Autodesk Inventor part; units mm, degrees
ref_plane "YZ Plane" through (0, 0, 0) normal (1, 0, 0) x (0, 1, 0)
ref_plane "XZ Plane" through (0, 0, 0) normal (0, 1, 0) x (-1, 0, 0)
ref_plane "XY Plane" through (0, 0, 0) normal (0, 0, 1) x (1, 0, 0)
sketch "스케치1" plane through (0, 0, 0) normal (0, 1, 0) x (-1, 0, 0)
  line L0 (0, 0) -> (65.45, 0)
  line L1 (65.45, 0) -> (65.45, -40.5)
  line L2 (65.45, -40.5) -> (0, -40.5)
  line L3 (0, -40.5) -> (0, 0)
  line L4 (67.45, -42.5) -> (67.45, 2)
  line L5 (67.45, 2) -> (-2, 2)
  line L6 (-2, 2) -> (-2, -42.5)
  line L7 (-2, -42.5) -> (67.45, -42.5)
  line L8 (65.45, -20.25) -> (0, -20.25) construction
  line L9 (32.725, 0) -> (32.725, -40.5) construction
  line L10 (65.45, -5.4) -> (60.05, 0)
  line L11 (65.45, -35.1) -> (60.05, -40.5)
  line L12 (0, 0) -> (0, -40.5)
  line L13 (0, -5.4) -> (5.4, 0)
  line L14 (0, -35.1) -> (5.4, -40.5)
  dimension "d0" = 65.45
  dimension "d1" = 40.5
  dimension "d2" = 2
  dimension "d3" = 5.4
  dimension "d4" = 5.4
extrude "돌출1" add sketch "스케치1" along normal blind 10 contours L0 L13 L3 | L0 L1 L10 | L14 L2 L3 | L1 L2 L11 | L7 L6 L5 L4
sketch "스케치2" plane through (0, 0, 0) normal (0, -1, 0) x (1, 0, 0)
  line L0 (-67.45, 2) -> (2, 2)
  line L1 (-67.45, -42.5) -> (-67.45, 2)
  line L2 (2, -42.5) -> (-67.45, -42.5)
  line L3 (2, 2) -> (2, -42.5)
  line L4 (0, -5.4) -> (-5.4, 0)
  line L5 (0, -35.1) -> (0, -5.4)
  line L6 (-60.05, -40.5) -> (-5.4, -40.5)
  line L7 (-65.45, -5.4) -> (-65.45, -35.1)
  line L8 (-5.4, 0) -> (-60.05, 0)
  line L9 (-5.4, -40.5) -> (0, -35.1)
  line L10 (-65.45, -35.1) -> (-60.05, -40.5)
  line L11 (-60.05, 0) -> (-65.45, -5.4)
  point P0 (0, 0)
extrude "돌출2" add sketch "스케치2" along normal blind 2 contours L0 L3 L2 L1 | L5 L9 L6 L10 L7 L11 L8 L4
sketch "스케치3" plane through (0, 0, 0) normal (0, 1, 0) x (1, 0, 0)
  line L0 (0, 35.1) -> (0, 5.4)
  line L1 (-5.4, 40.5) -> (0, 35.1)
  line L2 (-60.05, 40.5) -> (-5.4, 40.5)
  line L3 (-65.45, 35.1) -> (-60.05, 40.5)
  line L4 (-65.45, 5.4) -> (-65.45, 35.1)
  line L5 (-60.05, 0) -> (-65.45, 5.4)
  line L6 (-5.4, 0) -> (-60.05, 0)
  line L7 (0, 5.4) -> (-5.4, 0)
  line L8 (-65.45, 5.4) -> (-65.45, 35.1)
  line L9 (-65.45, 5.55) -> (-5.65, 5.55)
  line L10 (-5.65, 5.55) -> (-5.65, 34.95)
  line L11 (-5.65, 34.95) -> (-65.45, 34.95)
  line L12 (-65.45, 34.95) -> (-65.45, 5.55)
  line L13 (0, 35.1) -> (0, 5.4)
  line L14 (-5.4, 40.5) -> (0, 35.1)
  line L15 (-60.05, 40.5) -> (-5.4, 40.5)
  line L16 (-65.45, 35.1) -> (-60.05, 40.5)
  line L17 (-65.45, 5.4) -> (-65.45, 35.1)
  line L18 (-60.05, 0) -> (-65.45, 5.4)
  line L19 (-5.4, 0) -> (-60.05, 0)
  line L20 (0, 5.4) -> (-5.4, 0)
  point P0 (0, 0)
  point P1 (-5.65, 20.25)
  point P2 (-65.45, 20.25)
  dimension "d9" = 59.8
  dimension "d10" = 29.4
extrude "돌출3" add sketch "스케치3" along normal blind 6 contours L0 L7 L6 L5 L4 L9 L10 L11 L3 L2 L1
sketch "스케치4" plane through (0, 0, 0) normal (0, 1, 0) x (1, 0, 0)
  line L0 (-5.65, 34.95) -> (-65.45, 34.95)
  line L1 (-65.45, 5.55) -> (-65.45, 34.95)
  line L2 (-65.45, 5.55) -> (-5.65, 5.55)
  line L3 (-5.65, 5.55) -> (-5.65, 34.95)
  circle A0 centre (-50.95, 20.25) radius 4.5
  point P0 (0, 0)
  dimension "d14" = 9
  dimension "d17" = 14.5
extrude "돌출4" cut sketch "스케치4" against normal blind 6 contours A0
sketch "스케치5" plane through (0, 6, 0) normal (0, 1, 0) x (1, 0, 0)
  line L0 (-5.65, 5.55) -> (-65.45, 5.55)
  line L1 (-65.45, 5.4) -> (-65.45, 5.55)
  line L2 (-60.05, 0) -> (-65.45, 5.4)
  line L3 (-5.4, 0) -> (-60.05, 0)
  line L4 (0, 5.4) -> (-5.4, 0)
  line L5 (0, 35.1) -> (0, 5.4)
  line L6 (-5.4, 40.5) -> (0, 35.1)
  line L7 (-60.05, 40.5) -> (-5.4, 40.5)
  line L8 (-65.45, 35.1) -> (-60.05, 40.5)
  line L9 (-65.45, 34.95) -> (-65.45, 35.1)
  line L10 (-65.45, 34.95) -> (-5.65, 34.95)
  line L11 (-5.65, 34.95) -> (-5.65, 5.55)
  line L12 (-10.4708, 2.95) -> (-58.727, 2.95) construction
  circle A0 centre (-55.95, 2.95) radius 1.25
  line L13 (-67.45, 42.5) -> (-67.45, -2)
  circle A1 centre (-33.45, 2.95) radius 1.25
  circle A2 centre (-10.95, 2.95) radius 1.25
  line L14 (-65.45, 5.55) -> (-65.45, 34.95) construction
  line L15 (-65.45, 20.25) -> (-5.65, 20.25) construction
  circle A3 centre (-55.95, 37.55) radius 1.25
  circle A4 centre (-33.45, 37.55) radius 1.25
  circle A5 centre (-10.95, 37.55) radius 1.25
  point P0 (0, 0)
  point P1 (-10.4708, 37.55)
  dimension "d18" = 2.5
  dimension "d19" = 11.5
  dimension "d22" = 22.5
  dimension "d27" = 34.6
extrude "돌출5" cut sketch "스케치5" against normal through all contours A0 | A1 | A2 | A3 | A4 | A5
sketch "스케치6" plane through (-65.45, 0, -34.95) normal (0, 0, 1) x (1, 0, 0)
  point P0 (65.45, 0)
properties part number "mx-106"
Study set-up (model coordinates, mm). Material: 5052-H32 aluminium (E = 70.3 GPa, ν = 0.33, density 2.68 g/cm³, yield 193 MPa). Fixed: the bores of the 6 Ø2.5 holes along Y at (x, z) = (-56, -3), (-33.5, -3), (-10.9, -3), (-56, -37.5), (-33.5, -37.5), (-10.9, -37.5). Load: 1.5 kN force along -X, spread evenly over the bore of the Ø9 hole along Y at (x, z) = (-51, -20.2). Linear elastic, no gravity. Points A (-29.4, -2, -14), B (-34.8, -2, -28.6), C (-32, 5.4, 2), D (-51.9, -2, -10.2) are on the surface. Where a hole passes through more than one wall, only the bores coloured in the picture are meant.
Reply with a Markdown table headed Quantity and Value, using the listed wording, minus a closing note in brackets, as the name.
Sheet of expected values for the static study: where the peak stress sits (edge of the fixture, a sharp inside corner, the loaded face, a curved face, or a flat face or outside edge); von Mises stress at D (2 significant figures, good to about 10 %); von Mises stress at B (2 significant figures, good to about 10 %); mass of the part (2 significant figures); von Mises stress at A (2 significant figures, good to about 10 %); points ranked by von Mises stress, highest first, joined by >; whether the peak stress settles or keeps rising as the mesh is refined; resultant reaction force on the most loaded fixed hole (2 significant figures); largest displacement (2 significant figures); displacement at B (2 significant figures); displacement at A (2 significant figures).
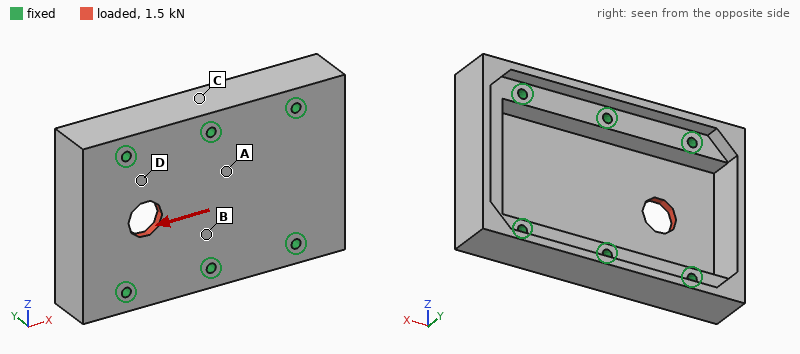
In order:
| Quantity | Value |
|---|---|
| where the peak stress sits | a sharp inside corner |
| von Mises stress at D | 16 MPa |
| von Mises stress at B | 11 MPa |
| mass of the part | 42 g |
| von Mises stress at A | 7.7 MPa |
| points ranked by von Mises stress, highest first, joined by > | D > B > A > C |
| whether the peak stress settles or keeps rising as the mesh is refined | keeps rising |
| resultant reaction force on the most loaded fixed hole | 380 N |
| largest displacement | 8.2 µm |
| displacement at B | 1.9 µm |
| displacement at A | 1.7 µm |
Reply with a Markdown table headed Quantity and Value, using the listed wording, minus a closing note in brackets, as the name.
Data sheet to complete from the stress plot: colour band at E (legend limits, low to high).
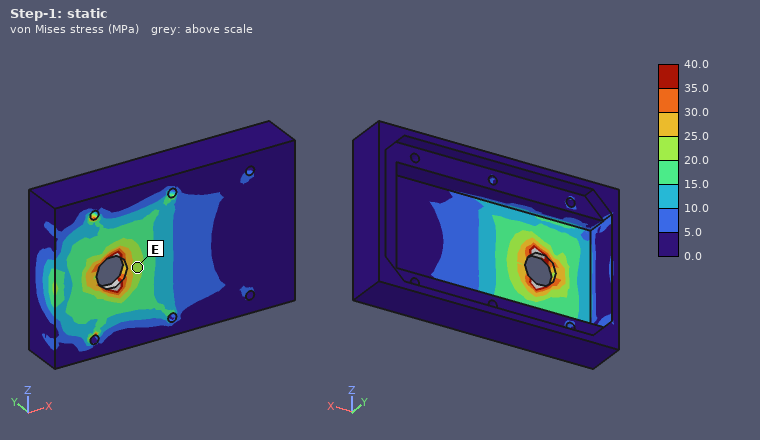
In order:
| Quantity | Value |
|---|---|
| colour band at E | 20.0 to 25.0 MPa |
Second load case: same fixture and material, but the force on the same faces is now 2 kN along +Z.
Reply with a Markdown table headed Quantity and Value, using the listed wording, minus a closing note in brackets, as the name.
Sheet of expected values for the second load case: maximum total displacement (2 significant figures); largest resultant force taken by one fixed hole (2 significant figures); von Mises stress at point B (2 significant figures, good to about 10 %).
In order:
| Quantity | Value |
|---|---|
| maximum total displacement | 6.9 µm |
| largest resultant force taken by one fixed hole | 700 N |
| von Mises stress at point B | 7.3 MPa |
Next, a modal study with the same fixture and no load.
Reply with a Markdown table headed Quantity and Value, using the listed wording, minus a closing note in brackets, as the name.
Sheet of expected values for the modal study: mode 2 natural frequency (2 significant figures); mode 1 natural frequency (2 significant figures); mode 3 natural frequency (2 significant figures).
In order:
| Quantity | Value |
|---|---|
| mode 2 natural frequency | 14 kHz |
| mode 1 natural frequency | 12 kHz |
| mode 3 natural frequency | 15 kHz |
